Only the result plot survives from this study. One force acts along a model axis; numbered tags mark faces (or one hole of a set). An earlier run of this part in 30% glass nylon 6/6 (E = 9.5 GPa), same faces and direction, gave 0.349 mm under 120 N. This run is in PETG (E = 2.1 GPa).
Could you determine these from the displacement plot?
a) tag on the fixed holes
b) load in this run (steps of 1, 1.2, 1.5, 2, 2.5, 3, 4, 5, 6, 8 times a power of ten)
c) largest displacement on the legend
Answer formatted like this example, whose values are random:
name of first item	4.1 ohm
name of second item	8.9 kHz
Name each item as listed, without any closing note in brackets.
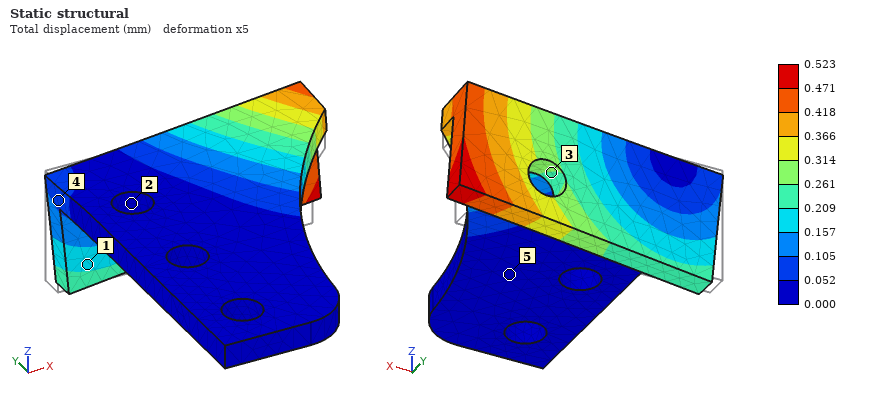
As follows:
tag on the fixed holes	2
load in this run	40 N
largest displacement on the legend	0.523 mm
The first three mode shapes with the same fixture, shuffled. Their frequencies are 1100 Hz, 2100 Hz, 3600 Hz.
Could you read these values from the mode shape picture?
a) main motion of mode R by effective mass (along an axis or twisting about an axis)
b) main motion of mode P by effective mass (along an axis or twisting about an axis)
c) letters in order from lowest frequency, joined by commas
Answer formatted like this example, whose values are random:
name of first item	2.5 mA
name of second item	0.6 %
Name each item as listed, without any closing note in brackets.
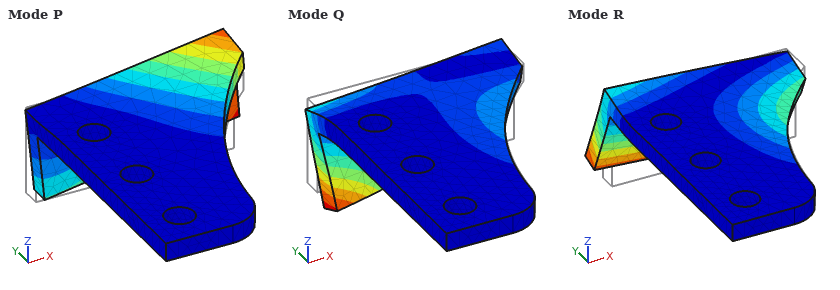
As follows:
main motion of mode R by effective mass	along Y
main motion of mode P by effective mass	along Z
letters in order from lowest frequency, joined by commas	P, R, Q
